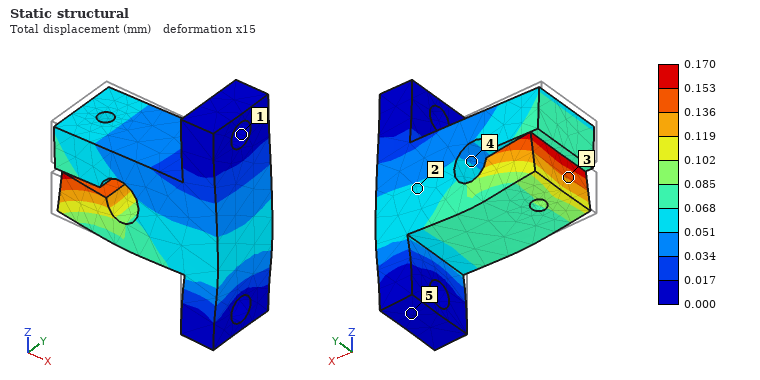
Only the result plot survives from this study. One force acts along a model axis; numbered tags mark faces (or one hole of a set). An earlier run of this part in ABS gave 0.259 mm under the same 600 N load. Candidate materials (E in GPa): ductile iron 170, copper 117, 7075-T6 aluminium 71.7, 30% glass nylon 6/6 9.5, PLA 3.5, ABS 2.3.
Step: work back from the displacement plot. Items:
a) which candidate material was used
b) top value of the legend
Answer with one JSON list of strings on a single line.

["PLA", "0.170 mm"]
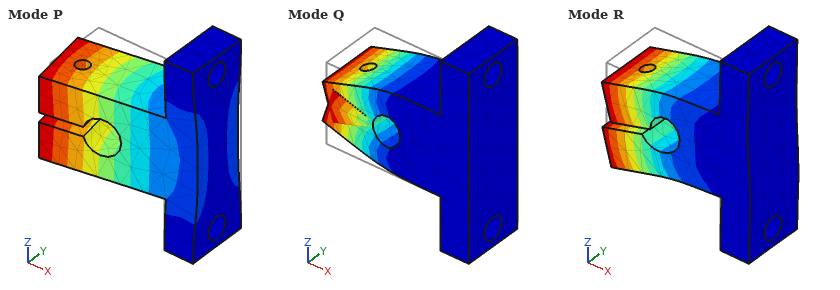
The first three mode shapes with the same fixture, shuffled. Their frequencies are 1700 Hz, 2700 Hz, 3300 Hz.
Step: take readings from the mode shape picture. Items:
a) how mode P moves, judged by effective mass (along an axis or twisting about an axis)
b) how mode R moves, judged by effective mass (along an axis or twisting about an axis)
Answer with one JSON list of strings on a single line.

["along Y", "along Z"]
